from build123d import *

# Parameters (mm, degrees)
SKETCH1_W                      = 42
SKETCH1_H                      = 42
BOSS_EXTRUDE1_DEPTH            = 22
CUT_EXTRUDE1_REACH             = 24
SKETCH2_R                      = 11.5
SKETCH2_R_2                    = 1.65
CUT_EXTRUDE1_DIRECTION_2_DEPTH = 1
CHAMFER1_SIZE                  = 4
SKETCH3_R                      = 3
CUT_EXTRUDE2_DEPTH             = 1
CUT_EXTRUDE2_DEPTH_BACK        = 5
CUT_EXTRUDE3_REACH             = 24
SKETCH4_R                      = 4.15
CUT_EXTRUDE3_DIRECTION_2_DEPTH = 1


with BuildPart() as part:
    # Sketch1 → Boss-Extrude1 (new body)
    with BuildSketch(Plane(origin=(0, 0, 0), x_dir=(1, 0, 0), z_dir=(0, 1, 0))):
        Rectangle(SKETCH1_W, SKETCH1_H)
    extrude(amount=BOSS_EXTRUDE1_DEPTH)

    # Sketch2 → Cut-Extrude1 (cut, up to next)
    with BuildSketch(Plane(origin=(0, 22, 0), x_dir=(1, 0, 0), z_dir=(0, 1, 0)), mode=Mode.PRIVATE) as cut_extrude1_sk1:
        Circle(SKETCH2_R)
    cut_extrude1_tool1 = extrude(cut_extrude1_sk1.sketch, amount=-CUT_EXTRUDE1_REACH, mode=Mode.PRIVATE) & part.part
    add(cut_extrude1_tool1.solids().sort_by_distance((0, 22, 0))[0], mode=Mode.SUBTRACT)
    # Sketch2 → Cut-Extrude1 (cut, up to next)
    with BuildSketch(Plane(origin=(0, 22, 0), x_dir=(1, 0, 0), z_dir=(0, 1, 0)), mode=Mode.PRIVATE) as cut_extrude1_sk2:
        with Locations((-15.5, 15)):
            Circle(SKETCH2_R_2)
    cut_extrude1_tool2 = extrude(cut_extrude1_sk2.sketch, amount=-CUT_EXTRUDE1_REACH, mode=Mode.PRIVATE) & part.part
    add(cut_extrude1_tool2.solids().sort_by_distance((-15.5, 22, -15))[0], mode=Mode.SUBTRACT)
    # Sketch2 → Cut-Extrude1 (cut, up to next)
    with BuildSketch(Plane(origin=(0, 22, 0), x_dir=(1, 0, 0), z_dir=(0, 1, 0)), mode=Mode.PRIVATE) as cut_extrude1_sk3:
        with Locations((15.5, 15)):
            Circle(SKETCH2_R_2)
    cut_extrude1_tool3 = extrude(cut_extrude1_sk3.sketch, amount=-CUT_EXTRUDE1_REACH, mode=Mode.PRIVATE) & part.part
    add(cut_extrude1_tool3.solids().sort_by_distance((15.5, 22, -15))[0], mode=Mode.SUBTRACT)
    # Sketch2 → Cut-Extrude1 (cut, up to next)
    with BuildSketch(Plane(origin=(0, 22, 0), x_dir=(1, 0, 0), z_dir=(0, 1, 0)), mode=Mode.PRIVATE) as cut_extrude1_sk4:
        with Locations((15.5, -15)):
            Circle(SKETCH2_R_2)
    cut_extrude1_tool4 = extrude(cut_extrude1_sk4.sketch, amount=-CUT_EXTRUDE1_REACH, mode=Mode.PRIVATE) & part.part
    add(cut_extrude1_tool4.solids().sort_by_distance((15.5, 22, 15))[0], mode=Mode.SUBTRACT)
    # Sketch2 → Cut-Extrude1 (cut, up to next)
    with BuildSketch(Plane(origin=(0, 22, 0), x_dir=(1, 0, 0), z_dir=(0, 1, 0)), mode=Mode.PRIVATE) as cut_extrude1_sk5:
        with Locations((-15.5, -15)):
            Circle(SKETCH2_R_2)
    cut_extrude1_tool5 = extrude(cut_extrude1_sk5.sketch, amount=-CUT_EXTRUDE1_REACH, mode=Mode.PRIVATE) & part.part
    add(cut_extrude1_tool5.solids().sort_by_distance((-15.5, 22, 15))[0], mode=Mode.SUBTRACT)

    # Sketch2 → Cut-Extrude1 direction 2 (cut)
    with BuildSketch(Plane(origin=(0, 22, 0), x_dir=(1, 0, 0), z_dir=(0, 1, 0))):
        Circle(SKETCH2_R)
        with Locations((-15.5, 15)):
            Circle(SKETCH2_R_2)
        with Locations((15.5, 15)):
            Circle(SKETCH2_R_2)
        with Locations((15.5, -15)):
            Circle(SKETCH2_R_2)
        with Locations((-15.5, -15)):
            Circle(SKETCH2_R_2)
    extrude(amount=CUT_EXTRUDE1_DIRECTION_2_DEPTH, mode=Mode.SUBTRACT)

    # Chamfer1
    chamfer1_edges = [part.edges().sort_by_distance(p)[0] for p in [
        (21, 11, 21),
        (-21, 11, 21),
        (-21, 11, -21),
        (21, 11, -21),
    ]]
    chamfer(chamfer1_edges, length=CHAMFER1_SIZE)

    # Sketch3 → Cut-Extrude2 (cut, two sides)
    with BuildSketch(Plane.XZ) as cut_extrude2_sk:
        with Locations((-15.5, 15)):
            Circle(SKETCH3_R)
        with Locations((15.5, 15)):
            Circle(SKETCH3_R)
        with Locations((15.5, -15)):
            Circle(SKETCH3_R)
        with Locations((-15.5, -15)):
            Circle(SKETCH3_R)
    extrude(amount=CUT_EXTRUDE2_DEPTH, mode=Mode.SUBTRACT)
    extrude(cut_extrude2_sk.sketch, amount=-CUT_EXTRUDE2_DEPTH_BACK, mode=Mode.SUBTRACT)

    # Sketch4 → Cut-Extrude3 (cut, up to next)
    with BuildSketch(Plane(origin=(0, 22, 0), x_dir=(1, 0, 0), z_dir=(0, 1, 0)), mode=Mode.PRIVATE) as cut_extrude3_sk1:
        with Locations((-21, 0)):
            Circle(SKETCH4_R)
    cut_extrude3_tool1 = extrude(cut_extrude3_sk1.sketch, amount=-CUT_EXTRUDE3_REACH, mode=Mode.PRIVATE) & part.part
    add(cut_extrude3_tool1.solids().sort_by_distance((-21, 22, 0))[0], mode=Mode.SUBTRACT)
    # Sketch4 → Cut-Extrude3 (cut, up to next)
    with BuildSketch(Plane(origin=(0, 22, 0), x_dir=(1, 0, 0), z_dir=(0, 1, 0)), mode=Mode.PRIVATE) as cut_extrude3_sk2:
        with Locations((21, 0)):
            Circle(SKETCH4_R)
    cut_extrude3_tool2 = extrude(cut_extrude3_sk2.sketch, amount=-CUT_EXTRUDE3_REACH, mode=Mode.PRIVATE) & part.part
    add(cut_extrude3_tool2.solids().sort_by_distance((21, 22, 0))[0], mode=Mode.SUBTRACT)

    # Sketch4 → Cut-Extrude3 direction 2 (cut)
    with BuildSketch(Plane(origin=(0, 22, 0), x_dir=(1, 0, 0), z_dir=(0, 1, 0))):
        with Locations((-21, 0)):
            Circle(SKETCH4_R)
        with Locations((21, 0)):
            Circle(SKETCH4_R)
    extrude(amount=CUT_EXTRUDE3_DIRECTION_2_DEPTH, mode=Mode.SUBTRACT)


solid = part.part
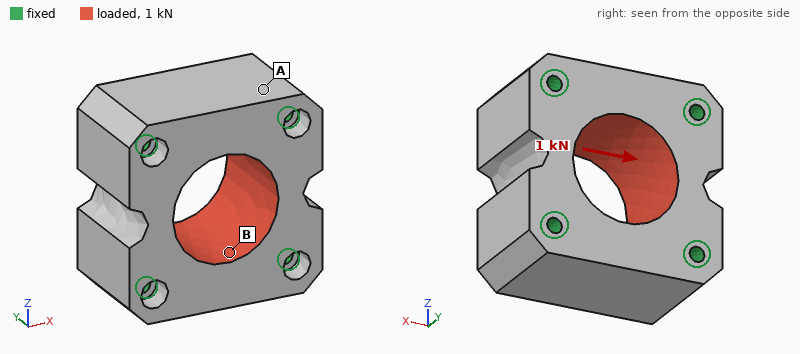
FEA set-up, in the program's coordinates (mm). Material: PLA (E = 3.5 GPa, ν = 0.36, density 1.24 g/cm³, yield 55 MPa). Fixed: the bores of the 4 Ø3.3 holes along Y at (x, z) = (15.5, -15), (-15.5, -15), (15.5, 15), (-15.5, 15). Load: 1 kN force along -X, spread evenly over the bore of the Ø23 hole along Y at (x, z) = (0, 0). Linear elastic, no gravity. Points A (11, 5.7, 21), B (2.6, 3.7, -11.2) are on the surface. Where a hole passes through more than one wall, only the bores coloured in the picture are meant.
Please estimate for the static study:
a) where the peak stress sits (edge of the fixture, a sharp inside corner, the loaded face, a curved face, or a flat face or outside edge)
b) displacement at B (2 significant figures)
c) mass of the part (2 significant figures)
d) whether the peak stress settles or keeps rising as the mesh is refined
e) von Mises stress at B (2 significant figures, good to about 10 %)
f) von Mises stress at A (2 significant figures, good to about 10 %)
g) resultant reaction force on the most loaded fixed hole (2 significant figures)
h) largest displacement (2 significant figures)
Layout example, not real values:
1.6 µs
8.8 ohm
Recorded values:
edge of the fixture
4.8 µm
33 g
keeps rising
1.3 MPa
0.58 MPa
270 N
13 µm
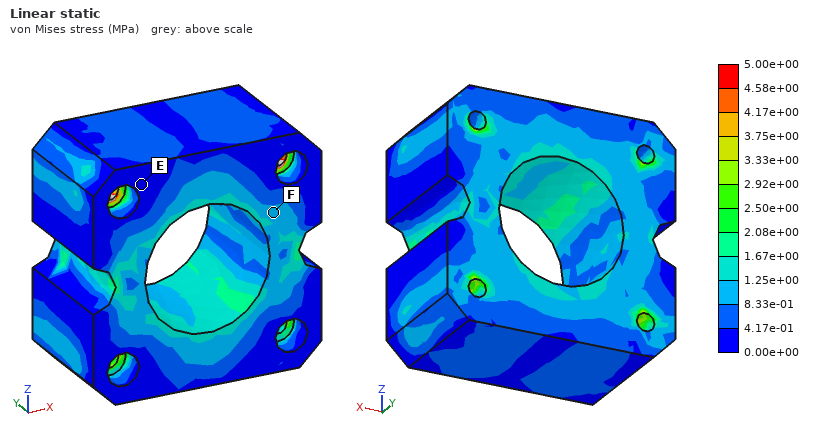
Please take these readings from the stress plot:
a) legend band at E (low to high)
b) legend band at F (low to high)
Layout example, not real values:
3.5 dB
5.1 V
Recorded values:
0.00e+00 to 4.17e-01 MPa
8.33e-01 to 1.25e+00 MPa
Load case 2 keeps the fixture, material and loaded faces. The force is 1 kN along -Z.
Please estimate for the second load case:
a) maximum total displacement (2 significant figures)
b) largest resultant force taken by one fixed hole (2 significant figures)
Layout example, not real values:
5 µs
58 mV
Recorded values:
12 µm
260 N
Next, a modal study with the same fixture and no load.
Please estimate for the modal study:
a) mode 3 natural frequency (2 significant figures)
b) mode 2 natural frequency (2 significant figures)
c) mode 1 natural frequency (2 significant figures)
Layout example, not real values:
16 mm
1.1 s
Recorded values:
12 kHz
12 kHz
8400 Hz
